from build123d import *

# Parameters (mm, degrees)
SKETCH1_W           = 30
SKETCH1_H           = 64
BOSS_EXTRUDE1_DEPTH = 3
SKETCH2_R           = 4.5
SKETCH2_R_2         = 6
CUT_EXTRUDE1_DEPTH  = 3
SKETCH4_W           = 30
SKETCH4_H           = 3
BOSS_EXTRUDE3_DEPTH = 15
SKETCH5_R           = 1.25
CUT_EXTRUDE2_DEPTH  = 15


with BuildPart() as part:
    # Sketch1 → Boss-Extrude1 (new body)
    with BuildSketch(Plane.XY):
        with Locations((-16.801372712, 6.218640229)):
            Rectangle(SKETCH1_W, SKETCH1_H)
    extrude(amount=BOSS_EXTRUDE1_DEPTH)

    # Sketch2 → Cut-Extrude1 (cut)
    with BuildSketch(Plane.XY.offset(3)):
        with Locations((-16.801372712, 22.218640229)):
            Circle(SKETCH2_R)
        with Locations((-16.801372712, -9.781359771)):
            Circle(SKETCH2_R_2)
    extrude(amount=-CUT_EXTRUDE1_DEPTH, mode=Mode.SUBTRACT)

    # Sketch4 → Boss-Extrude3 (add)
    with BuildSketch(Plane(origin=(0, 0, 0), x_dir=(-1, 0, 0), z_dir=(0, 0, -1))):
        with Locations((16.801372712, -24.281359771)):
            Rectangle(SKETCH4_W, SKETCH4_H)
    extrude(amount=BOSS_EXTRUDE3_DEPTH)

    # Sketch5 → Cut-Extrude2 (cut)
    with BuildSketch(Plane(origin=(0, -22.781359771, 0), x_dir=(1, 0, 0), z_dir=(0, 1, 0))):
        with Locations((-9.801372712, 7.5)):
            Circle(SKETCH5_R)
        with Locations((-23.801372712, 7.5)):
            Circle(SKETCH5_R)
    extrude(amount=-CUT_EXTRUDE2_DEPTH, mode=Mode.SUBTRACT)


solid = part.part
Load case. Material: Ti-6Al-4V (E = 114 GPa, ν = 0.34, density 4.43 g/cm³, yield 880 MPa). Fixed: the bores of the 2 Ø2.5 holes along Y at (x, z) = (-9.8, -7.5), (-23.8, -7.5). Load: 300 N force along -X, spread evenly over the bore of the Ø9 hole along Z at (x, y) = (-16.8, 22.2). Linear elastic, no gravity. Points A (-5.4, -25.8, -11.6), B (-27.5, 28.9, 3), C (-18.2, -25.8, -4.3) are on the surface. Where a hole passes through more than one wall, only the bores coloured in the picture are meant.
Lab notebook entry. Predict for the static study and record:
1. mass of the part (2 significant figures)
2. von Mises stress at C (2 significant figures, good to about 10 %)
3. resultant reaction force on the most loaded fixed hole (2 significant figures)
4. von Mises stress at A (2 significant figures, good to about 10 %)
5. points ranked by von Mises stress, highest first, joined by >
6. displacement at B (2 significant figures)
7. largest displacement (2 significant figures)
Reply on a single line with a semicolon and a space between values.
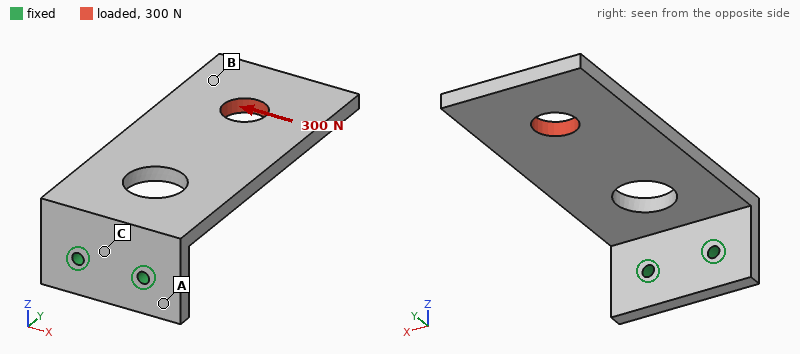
29 g; 78 MPa; 810 N; 50 MPa; C > A > B; 0.22 mm; 0.27 mm
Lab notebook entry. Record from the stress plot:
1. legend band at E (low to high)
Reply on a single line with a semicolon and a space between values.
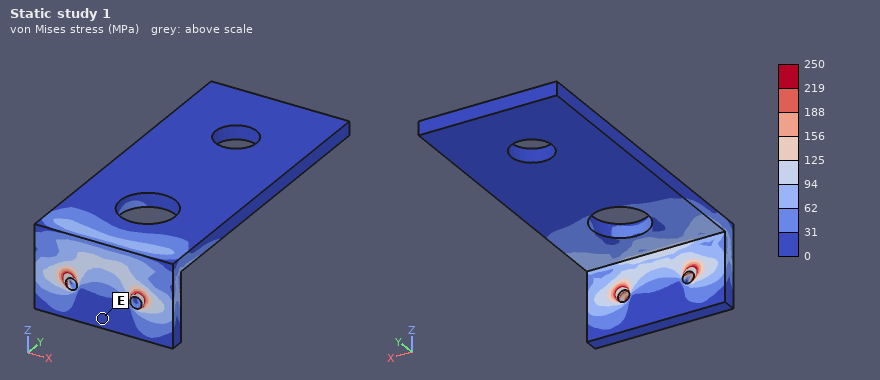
0 to 31 MPa
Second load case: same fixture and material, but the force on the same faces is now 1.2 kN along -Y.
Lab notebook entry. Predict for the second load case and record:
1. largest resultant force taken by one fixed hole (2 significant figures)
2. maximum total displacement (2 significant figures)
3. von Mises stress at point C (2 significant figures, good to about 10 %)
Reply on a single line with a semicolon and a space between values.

600 N; 0.44 mm; 110 MPa
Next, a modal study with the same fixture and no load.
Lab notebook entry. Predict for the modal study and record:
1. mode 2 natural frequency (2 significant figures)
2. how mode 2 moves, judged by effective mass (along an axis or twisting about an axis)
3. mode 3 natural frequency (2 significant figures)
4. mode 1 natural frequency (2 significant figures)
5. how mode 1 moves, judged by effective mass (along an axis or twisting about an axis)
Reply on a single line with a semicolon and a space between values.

1600 Hz; along X; 2500 Hz; 490 Hz; along Z
